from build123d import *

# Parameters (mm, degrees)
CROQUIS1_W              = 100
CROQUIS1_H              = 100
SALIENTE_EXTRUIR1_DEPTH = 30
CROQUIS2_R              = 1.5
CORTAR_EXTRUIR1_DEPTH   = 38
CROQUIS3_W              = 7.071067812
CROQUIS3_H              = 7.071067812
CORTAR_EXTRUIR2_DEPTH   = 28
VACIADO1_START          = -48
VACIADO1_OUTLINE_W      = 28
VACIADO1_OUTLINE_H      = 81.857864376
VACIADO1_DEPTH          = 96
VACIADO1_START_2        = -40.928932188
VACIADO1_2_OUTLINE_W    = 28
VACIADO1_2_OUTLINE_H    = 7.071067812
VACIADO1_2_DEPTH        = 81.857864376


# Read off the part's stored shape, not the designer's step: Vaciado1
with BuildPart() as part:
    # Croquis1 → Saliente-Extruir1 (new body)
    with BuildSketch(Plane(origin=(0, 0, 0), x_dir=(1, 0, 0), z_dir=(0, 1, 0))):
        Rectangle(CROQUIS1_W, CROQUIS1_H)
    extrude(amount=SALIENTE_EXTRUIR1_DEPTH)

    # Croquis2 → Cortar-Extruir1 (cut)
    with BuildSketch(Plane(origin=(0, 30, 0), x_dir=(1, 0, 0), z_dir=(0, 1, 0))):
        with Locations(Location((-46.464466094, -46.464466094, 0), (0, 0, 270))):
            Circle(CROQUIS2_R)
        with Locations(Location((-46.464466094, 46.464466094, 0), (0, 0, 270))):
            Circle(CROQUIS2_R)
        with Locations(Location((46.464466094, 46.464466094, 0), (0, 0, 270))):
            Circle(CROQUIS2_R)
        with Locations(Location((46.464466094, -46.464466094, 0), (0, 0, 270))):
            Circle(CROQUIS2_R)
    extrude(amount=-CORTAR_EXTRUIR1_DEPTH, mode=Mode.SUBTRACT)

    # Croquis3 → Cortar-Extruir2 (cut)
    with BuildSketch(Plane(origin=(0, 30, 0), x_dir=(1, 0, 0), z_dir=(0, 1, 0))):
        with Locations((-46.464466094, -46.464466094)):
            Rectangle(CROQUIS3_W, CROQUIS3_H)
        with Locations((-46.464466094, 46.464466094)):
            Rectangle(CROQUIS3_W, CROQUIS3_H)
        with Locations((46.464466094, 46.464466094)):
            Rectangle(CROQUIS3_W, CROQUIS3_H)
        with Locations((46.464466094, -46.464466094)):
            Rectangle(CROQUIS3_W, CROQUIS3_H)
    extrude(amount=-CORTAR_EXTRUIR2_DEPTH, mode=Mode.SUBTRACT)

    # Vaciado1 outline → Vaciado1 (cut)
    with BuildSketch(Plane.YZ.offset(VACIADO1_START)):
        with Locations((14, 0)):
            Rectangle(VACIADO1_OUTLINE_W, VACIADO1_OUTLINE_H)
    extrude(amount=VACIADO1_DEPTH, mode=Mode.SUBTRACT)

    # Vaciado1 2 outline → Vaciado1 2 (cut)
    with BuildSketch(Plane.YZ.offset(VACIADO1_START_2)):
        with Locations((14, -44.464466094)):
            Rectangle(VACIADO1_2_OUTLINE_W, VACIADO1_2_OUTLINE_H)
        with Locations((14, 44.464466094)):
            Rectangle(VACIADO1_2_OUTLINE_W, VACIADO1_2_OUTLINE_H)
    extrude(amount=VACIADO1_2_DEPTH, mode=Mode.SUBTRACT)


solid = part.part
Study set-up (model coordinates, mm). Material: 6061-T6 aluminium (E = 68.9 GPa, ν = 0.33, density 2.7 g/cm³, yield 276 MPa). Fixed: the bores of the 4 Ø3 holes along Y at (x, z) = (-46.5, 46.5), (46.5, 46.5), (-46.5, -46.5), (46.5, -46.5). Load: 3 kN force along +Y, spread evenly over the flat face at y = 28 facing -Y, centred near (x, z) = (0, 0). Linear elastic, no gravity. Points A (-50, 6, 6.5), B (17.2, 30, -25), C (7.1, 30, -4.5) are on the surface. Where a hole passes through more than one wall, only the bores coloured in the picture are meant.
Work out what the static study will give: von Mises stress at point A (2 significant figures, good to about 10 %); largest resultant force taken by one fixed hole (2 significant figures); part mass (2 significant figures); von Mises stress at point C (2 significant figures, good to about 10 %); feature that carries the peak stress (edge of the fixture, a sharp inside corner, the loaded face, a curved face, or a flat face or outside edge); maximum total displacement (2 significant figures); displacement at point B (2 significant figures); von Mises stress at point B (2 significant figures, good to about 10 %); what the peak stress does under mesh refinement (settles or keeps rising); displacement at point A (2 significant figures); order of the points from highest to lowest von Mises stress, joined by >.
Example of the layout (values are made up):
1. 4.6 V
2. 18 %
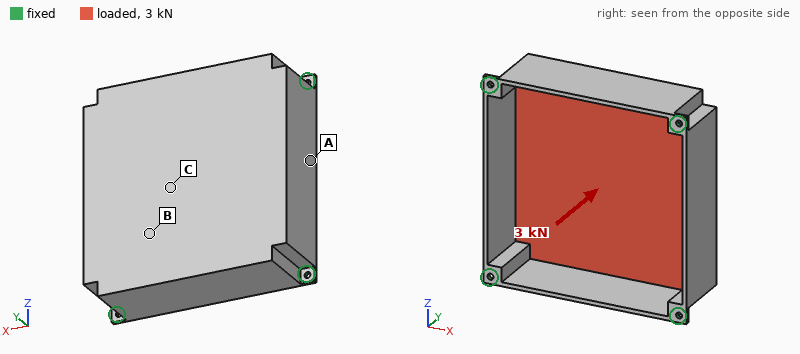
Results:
1. 56 MPa
2. 830 N
3. 110 g
4. 150 MPa
5. edge of the fixture
6. 1.2 mm
7. 0.67 mm
8. 91 MPa
9. keeps rising
10. 0.33 mm
11. C > B > A
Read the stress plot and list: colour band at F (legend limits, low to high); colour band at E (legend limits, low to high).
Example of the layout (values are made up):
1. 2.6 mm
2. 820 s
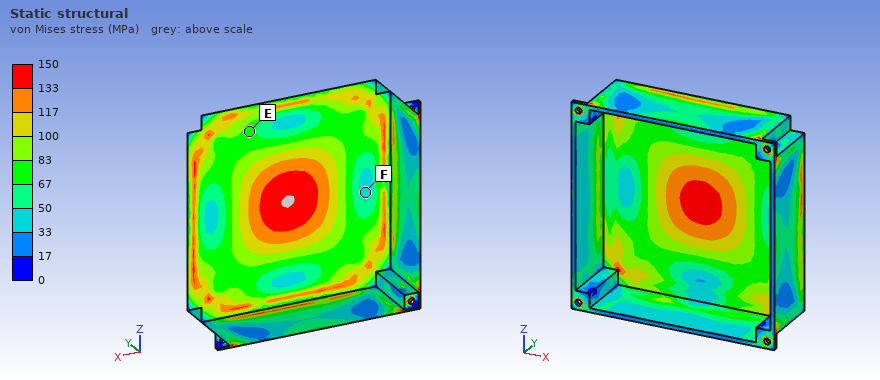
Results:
1. 33 to 50 MPa
2. 67 to 83 MPa
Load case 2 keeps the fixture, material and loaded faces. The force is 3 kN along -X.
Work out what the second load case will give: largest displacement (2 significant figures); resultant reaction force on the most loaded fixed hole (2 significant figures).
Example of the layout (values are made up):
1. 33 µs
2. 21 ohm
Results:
1. 41 µm
2. 870 N
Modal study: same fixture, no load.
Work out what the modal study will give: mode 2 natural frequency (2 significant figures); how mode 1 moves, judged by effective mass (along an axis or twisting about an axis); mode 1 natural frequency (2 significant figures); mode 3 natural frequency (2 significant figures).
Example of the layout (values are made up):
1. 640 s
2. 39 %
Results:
1. 2300 Hz
2. along Y
3. 1400 Hz
4. 2300 Hz
